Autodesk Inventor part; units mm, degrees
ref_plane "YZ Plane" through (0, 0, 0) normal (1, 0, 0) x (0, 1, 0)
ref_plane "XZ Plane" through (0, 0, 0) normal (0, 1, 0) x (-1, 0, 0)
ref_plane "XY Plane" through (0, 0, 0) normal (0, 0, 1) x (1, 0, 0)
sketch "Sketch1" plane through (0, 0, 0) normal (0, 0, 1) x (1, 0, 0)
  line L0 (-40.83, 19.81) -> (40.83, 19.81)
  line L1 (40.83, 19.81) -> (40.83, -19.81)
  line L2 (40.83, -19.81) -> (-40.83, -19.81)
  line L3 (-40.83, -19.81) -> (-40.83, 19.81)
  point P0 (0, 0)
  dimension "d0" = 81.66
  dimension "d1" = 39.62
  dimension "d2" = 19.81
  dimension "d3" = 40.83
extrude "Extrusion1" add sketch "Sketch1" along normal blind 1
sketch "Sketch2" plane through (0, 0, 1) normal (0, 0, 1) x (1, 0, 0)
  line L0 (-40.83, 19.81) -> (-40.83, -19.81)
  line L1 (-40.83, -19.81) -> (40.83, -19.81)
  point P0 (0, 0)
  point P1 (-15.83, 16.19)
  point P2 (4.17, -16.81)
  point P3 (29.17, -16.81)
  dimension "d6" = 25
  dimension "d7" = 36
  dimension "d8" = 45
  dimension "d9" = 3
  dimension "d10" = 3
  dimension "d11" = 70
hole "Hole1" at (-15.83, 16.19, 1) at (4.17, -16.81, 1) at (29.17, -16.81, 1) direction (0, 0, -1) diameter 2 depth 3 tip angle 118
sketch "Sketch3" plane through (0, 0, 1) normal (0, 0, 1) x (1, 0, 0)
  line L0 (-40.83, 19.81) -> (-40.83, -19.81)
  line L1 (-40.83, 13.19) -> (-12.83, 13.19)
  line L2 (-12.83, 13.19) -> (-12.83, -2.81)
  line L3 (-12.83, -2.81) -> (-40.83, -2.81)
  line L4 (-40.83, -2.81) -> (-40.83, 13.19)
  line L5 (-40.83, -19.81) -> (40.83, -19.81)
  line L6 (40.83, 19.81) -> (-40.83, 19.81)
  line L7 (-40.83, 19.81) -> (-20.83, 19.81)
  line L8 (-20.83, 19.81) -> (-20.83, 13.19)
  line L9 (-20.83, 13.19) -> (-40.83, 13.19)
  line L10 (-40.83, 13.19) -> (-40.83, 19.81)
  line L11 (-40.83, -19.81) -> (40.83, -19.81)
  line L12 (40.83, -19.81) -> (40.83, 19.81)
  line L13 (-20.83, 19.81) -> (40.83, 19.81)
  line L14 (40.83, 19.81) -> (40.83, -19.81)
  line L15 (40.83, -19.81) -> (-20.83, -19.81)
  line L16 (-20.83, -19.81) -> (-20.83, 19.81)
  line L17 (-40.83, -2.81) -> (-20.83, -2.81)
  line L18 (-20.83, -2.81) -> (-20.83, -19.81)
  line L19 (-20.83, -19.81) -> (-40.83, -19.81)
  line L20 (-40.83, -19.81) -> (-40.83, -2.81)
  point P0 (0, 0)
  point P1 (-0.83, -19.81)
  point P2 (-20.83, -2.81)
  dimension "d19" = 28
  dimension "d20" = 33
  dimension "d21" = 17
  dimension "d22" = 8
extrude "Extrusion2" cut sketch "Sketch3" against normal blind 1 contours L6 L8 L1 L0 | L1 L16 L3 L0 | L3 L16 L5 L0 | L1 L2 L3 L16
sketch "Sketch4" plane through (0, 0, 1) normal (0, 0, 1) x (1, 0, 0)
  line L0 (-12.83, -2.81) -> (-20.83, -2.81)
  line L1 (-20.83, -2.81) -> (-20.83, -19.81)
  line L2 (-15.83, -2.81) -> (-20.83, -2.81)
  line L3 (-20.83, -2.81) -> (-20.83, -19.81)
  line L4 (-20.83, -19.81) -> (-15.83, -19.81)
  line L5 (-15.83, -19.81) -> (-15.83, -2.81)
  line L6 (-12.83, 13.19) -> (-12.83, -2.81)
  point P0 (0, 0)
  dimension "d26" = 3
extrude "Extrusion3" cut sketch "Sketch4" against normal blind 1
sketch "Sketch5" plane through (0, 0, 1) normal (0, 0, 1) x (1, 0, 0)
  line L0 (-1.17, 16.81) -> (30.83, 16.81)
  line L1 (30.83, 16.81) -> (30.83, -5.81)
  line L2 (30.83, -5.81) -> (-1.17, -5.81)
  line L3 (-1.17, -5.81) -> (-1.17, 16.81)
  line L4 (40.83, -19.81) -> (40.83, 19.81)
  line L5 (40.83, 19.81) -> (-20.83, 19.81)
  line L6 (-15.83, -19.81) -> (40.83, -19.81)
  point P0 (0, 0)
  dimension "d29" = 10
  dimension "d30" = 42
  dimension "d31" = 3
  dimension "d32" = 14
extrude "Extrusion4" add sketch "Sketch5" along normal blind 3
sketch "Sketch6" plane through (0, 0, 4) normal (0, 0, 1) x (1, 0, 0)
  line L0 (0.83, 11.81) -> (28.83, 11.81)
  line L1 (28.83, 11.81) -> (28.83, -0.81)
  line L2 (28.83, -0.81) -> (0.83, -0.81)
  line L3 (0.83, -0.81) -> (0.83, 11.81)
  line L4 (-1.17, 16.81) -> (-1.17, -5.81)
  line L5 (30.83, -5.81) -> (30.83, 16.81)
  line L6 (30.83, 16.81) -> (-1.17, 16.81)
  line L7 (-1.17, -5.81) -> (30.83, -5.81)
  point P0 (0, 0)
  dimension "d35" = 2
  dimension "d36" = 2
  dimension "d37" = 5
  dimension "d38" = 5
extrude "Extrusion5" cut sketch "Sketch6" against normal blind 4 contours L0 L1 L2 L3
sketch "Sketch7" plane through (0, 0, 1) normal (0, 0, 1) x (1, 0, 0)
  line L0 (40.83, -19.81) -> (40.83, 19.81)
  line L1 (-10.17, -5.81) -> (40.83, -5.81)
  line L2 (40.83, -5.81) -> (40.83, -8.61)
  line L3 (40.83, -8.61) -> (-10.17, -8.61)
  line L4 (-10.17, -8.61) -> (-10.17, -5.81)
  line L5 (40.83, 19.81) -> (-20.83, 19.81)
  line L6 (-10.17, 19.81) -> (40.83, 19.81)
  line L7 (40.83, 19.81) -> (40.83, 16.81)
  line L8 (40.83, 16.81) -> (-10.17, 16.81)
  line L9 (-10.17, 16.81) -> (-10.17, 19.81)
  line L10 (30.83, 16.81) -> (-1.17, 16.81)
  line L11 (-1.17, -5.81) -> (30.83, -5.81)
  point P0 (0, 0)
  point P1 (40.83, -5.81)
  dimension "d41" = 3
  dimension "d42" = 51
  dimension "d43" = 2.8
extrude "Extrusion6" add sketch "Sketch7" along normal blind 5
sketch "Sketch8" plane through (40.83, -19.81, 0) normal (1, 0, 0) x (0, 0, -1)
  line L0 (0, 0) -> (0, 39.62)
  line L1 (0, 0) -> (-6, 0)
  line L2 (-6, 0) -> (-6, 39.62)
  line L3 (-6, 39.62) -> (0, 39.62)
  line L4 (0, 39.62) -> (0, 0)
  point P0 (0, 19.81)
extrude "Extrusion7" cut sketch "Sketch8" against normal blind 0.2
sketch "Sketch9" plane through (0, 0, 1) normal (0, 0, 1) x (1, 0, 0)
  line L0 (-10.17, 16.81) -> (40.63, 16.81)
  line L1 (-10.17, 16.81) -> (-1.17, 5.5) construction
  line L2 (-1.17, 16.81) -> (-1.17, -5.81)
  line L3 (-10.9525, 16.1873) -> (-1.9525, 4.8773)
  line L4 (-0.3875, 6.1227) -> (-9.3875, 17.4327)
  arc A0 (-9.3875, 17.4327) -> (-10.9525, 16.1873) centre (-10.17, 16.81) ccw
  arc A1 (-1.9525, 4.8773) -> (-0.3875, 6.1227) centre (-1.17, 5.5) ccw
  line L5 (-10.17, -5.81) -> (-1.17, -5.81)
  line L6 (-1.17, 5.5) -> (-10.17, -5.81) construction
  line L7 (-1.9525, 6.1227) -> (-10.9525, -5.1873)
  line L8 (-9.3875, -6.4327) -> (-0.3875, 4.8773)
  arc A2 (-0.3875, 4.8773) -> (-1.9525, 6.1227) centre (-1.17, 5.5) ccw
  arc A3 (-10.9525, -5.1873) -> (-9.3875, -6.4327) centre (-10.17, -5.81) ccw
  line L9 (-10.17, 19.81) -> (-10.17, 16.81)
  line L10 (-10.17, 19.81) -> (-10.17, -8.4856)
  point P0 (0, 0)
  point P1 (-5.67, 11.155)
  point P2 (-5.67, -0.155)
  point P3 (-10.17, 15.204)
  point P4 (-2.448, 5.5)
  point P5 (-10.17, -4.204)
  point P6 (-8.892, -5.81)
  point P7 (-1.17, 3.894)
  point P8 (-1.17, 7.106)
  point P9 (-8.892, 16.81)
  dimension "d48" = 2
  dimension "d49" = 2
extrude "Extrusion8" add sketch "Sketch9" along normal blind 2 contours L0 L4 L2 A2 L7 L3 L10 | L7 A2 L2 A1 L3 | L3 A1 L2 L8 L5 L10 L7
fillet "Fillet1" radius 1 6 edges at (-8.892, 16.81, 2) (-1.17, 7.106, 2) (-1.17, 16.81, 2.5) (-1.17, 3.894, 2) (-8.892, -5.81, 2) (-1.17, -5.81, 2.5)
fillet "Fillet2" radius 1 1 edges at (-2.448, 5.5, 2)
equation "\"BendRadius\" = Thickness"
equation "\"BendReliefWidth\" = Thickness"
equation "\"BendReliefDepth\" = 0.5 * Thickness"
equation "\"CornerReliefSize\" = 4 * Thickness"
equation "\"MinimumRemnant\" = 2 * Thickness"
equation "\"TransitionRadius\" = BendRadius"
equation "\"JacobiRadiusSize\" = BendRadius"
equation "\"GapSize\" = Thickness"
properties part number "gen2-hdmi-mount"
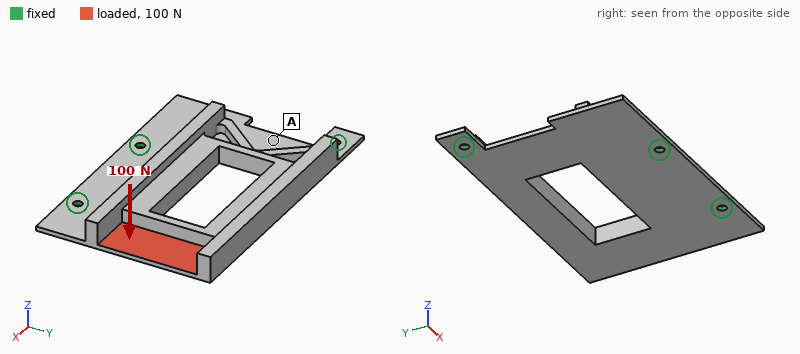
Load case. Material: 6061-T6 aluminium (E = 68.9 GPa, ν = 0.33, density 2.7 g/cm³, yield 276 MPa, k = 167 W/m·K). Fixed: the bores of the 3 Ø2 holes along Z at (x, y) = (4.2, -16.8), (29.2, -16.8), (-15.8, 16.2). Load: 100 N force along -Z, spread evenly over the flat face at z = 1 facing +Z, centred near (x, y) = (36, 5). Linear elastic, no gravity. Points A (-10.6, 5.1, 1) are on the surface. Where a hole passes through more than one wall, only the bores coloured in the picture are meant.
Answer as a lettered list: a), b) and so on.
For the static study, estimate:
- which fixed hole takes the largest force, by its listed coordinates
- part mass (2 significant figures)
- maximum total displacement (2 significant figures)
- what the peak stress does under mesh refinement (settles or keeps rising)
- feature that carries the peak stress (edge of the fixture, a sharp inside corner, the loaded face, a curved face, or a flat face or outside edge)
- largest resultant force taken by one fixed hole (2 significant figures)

a) (29.2, -16.8)
b) 12 g
c) 0.85 mm
d) keeps rising
e) edge of the fixture
f) 200 N
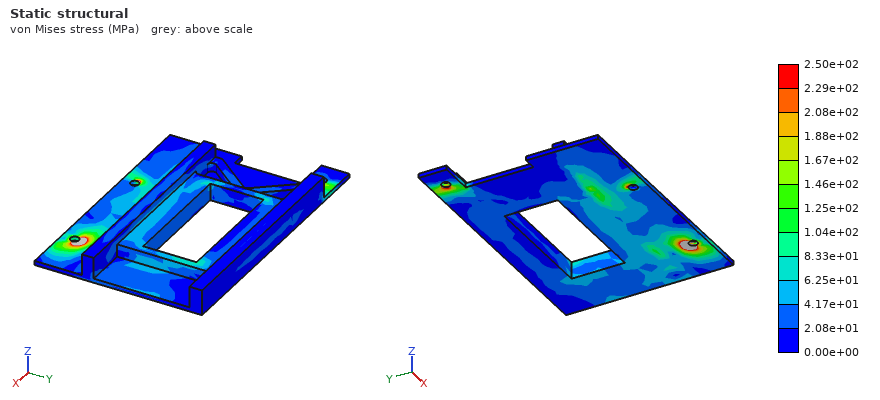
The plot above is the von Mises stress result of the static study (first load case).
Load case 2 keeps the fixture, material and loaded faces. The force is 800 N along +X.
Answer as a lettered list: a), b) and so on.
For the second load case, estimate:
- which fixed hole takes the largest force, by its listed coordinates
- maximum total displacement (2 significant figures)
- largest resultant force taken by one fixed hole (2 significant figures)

a) (-15.8, 16.2)
b) 70 µm
c) 380 N
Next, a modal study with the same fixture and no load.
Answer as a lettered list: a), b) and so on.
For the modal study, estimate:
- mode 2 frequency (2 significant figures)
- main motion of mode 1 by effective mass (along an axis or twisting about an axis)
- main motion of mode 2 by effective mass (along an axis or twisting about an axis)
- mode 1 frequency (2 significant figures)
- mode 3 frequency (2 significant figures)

a) 3500 Hz
b) along Z
c) along Z
d) 1000 Hz
e) 4600 Hz
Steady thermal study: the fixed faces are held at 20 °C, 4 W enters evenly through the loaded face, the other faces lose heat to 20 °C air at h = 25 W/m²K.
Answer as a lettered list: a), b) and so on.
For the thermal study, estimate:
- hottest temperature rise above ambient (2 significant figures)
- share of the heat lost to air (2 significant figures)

a) 14 K
b) 17 %
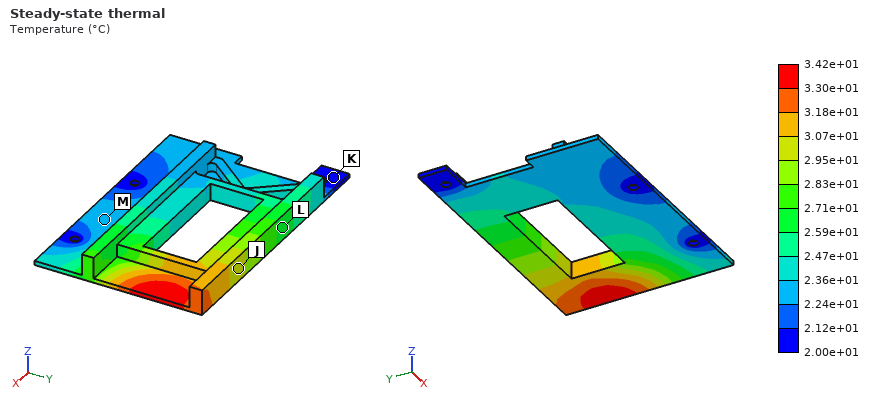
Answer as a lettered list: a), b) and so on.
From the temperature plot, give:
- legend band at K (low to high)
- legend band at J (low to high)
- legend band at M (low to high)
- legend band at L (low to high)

a) 2.00e+01 to 2.12e+01 °C
b) 2.95e+01 to 3.07e+01 °C
c) 2.24e+01 to 2.36e+01 °C
d) 2.59e+01 to 2.71e+01 °C
